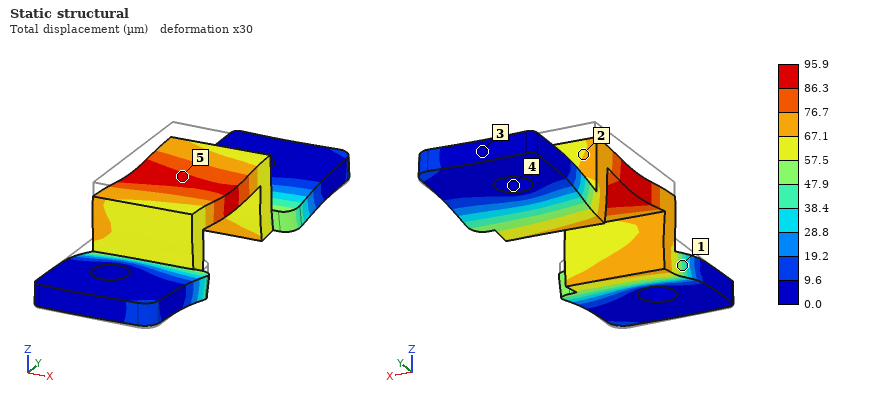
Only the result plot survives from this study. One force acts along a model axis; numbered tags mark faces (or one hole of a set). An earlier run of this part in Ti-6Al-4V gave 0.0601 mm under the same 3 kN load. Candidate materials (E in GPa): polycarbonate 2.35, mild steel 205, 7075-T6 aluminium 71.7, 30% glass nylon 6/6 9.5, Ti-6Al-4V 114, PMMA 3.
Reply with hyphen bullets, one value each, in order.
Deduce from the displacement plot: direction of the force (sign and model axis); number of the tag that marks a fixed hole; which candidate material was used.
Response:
- -Z
- 4
- 7075-T6 aluminium
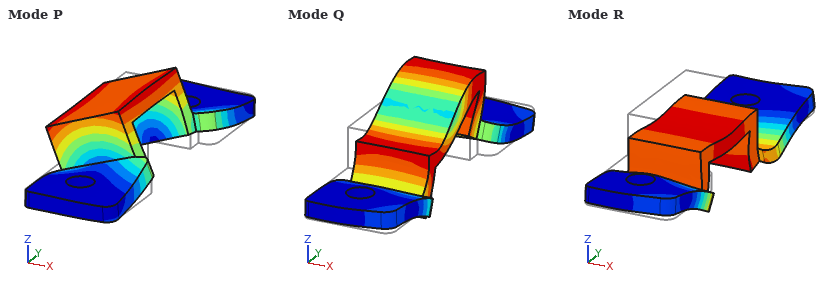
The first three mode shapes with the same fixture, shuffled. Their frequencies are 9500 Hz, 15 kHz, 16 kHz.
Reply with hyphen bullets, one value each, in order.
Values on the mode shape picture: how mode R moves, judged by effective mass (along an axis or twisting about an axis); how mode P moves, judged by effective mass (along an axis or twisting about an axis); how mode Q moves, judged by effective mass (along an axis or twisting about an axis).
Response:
- along Z
- along X
- along Y
